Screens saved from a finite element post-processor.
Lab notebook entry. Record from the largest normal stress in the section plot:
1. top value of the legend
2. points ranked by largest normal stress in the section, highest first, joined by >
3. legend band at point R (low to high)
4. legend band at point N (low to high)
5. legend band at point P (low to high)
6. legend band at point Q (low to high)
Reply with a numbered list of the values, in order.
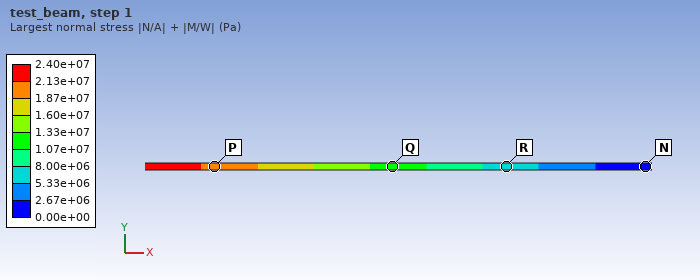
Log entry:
1. 2.40e+07 Pa
2. P > Q > R > N
3. 5.33e+06 to 8.00e+06 Pa
4. 0.00e+00 to 2.67e+06 Pa
5. 1.87e+07 to 2.13e+07 Pa
6. 1.07e+07 to 1.33e+07 Pa
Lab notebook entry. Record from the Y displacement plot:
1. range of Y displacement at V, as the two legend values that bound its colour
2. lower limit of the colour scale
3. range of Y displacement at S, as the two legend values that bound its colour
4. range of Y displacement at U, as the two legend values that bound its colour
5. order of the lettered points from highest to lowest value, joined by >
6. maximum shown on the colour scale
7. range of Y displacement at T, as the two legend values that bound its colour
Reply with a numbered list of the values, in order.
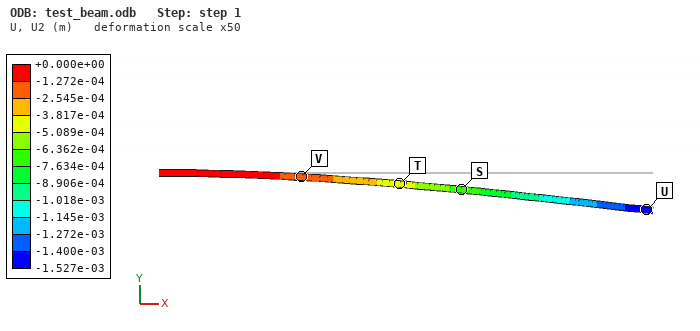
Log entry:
1. -2.545e-04 to -1.272e-04 m
2. -1.527e-03 m
3. -7.634e-04 to -6.362e-04 m
4. -1.527e-03 to -1.400e-03 m
5. V > T > S > U
6. +0.000e+00 m
7. -5.089e-04 to -3.817e-04 m
